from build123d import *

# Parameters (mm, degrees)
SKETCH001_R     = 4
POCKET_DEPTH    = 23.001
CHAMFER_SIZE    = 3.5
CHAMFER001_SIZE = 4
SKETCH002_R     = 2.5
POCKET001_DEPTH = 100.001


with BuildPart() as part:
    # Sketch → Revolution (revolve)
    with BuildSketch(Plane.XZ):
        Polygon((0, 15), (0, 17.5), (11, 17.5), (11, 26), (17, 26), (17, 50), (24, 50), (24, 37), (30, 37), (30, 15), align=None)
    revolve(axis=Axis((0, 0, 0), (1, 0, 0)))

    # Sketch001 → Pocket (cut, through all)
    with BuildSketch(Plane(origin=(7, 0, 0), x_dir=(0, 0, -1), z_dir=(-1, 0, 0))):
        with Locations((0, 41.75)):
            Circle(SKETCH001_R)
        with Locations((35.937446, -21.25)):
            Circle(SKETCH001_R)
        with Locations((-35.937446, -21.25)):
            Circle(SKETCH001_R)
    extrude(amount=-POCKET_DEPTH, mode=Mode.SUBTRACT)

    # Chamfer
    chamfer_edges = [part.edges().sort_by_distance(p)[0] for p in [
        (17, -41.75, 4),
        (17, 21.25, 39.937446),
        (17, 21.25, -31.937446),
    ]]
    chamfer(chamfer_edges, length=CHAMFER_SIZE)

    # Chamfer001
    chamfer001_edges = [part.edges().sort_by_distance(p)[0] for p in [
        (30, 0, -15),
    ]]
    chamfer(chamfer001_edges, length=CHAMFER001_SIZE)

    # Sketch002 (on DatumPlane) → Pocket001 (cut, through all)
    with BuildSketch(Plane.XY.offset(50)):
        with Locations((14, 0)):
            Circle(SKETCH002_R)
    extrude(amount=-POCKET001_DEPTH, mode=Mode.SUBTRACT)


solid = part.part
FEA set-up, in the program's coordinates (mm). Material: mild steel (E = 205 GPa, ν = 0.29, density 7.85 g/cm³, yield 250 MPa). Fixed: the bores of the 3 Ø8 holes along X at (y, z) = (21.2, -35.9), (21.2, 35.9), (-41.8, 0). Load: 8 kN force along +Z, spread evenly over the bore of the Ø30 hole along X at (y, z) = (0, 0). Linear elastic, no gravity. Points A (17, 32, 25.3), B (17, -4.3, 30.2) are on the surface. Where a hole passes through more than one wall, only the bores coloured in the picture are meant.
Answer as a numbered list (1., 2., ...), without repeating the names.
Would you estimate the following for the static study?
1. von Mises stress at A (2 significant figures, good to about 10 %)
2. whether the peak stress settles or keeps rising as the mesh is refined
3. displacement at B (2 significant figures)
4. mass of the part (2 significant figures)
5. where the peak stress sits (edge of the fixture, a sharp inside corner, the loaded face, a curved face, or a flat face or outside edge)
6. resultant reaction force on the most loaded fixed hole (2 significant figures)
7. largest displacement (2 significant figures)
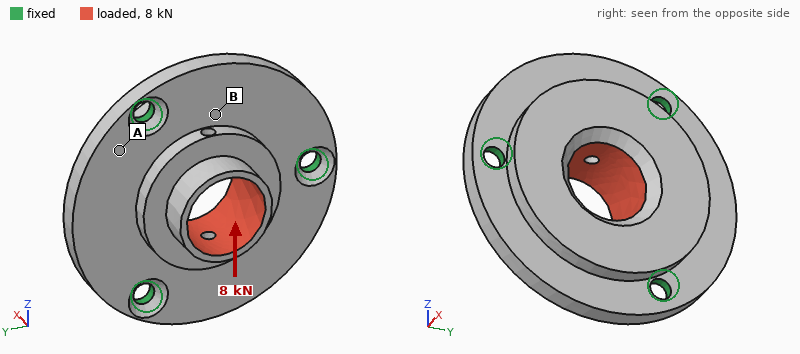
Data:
1. 7.6 MPa
2. keeps rising
3. 5.3 µm
4. 630 g
5. edge of the fixture
6. 2.8 kN
7. 12 µm
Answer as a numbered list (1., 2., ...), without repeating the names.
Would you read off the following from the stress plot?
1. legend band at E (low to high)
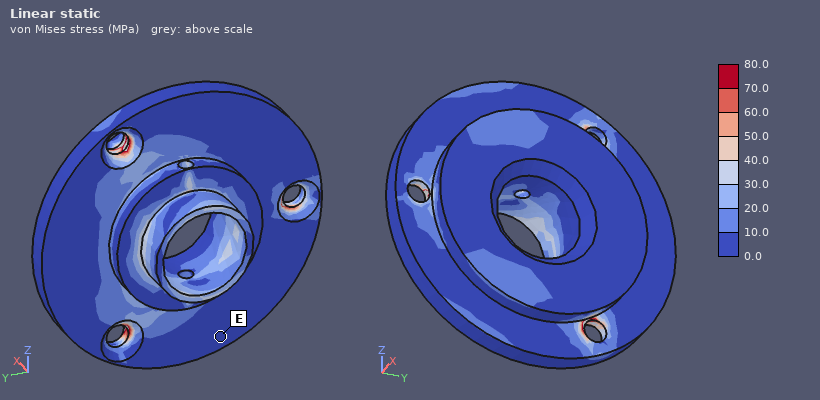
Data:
1. 0.0 to 10.0 MPa
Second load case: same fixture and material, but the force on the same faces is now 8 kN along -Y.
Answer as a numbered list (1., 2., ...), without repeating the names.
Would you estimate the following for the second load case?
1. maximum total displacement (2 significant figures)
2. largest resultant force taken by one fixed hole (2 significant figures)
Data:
1. 13 µm
2. 2.9 kN
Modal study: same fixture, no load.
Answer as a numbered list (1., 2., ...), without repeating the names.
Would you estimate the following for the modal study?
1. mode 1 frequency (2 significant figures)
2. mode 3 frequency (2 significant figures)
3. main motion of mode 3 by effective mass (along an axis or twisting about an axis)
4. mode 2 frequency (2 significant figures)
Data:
1. 5500 Hz
2. 6400 Hz
3. along X
4. 5600 Hz
